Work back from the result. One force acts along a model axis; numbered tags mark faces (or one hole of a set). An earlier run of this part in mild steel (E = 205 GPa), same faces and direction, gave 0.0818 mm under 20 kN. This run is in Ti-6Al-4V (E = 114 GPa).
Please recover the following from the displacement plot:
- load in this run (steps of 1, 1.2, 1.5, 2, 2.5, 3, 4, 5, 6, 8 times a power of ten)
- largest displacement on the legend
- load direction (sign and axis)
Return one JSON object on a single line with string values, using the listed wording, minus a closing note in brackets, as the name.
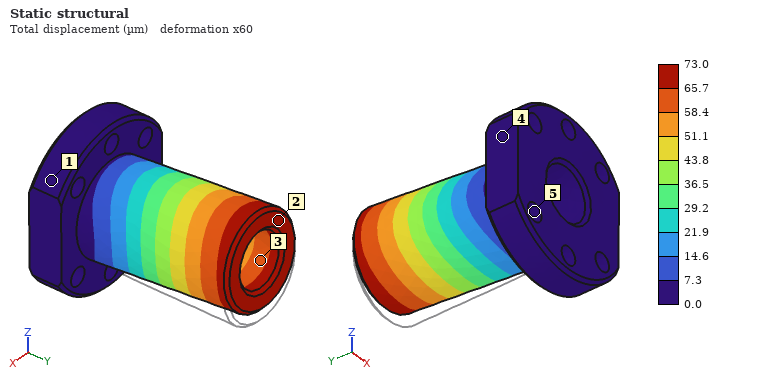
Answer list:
{"load in this run": "10 kN", "largest displacement on the legend": "73.0 µm", "load direction": "+Z"}
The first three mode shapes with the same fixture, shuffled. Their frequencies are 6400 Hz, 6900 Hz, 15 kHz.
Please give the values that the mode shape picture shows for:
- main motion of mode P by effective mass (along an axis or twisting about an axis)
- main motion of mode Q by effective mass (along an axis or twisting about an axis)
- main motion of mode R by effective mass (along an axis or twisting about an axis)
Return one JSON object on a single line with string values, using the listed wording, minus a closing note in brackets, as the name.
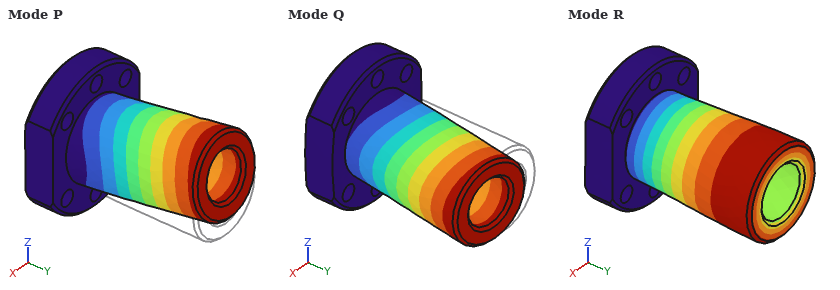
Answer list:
{"main motion of mode P by effective mass": "along Z", "main motion of mode Q by effective mass": "along X", "main motion of mode R by effective mass": "twisting about Y"}
